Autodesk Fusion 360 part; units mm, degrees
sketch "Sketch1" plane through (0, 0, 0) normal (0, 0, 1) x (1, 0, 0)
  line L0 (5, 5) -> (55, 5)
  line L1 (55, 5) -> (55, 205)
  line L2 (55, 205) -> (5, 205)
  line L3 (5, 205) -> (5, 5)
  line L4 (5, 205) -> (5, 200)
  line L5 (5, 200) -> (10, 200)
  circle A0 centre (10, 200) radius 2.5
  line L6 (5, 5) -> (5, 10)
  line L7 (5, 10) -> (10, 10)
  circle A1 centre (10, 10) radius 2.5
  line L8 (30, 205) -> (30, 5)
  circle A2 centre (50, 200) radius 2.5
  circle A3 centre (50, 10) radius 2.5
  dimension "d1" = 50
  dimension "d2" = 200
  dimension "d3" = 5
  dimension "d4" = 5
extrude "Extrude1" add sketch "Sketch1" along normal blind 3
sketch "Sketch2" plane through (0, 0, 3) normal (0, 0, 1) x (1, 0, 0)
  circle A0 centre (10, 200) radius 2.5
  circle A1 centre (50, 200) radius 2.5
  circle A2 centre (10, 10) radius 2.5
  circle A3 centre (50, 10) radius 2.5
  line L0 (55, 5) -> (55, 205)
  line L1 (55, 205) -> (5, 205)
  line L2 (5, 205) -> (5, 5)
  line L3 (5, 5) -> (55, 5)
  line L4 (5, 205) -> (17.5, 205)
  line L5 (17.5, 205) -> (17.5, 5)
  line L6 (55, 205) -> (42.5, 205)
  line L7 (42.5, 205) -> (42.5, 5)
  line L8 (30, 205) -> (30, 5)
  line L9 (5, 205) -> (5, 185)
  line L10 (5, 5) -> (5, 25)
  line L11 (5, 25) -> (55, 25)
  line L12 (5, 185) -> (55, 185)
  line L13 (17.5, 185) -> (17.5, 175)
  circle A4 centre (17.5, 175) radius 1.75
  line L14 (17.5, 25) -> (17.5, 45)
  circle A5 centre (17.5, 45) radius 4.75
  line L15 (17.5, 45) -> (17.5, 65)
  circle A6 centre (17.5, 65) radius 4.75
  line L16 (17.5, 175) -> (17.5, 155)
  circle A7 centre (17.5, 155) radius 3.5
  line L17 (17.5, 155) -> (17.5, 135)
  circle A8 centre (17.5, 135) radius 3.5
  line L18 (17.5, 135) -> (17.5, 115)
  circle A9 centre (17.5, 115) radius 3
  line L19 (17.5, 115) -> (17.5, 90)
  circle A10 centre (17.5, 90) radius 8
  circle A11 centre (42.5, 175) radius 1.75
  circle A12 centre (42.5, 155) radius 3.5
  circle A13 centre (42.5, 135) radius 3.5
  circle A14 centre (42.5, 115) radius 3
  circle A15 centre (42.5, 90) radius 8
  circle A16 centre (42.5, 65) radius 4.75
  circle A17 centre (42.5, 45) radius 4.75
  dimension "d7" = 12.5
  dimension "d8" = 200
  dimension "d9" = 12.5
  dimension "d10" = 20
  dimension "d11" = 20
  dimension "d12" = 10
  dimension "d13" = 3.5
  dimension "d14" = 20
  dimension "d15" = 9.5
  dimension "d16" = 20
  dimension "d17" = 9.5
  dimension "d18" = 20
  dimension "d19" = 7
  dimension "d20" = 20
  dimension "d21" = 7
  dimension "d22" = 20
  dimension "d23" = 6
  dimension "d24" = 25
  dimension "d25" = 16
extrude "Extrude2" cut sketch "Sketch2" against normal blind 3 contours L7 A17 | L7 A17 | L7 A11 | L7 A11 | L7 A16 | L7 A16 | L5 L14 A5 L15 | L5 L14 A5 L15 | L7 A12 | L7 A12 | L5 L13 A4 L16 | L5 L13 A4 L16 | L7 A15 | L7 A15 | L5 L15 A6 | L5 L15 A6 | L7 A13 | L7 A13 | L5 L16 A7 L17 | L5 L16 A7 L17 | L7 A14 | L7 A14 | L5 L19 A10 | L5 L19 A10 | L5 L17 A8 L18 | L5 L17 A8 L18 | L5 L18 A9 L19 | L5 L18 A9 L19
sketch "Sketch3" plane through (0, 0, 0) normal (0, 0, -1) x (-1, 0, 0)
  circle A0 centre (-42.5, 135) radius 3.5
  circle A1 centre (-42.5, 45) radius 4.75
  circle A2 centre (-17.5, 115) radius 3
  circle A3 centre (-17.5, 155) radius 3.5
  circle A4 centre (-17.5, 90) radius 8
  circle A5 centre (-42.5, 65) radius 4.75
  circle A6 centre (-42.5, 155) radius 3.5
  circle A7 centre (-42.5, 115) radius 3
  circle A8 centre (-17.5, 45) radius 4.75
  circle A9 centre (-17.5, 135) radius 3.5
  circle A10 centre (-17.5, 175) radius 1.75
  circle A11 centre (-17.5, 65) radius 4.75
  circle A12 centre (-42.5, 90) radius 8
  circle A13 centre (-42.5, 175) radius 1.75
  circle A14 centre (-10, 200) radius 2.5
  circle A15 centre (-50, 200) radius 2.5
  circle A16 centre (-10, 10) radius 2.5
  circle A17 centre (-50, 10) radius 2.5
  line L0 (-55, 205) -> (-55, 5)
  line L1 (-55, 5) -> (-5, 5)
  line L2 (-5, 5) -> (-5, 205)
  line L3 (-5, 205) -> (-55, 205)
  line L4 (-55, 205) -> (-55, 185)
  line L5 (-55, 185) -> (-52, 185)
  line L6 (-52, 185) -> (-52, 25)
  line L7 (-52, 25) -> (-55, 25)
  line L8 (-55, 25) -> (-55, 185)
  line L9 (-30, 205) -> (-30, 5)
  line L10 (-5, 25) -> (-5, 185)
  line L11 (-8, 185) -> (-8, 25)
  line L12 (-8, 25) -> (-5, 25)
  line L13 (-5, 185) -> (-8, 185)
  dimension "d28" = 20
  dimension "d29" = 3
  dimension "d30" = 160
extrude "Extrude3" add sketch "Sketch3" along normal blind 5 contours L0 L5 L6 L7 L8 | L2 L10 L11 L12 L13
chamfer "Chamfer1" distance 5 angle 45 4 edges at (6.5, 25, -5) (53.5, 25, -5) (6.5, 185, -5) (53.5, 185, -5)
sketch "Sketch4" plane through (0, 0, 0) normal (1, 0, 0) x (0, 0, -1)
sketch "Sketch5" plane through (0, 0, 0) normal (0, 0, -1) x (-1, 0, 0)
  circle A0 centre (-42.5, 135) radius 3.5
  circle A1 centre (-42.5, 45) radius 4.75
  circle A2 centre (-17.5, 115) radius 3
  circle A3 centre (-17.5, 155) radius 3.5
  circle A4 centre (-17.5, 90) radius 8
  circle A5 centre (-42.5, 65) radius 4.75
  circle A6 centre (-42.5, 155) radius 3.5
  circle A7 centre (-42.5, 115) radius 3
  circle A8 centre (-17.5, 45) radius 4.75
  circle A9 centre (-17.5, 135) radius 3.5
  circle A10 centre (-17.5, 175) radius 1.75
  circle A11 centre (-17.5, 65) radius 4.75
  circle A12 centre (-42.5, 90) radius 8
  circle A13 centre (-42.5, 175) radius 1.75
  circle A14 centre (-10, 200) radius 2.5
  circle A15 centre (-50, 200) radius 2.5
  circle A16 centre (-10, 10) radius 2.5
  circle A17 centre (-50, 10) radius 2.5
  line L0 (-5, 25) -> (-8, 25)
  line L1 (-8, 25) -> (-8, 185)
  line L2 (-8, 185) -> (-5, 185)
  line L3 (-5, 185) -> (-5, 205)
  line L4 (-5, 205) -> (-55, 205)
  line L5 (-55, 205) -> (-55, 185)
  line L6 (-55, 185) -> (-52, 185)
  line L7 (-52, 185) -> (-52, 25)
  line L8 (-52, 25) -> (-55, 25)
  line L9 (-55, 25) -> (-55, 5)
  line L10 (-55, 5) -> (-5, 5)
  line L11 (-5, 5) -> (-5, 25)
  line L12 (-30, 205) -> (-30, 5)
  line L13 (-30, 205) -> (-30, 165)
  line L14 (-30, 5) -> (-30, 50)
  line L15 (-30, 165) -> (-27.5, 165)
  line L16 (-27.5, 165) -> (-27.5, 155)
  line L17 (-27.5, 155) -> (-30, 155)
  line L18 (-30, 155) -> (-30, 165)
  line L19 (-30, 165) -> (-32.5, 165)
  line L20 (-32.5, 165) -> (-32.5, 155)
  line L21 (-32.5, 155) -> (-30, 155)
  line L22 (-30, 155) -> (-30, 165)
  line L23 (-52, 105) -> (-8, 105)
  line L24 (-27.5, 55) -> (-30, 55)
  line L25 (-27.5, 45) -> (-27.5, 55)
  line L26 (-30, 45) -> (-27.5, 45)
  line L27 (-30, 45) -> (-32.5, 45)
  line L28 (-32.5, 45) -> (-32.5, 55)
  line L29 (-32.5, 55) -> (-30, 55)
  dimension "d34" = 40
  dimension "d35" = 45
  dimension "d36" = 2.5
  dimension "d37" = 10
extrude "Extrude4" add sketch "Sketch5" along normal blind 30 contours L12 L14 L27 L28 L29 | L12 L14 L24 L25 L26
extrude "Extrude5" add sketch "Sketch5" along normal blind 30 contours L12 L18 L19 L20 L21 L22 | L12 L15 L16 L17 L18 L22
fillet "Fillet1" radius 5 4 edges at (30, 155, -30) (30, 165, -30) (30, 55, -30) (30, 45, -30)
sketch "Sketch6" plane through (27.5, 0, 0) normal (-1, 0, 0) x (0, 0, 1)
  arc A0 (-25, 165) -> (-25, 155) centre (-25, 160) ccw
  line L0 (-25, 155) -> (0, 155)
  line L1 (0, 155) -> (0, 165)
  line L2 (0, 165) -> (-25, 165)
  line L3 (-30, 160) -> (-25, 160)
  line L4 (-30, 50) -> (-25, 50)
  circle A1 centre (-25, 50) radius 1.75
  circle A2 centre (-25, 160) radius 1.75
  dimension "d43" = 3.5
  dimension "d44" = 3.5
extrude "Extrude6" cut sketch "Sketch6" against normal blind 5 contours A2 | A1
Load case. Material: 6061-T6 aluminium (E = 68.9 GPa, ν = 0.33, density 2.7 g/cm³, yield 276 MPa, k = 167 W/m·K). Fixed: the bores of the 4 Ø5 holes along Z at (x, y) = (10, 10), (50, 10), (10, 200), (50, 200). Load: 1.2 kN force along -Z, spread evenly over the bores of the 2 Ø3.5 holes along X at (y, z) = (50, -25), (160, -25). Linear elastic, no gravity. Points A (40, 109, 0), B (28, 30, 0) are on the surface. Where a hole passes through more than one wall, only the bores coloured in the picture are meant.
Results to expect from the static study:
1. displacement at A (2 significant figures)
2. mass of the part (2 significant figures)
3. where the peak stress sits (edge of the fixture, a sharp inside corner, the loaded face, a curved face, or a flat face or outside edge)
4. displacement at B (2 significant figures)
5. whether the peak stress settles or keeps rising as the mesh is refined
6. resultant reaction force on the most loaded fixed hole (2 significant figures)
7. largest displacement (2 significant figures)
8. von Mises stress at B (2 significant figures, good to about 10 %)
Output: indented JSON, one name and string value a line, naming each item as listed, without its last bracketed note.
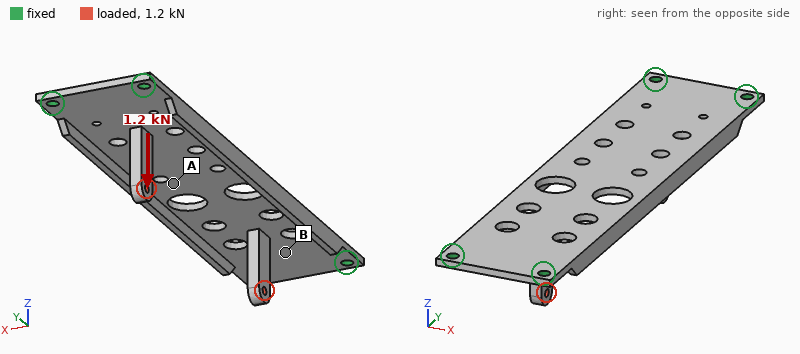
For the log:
{
  "displacement at A": "1.0 mm",
  "mass of the part": "93 g",
  "where the peak stress sits": "edge of the fixture",
  "displacement at B": "0.28 mm",
  "whether the peak stress settles or keeps rising as the mesh is refined": "keeps rising",
  "resultant reaction force on the most loaded fixed hole": "790 N",
  "largest displacement": "1.0 mm",
  "von Mises stress at B": "44 MPa"
}
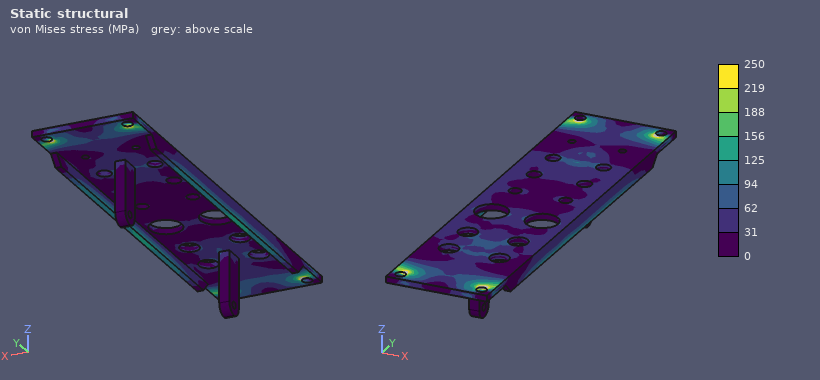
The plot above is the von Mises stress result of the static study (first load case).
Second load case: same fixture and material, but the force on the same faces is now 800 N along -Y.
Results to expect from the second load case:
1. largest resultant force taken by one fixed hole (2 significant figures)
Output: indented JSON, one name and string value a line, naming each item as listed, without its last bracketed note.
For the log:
{
  "largest resultant force taken by one fixed hole": "240 N"
}
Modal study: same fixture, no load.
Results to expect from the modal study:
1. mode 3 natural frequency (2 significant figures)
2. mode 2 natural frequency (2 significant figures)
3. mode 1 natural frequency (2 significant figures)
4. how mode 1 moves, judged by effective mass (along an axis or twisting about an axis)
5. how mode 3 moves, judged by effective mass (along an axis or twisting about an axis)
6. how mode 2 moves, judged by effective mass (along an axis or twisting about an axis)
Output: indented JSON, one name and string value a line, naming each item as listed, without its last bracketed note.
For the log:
{
  "mode 3 natural frequency": "1700 Hz",
  "mode 2 natural frequency": "1100 Hz",
  "mode 1 natural frequency": "610 Hz",
  "how mode 1 moves, judged by effective mass": "along Z",
  "how mode 3 moves, judged by effective mass": "twisting about X",
  "how mode 2 moves, judged by effective mass": "twisting about Y"
}
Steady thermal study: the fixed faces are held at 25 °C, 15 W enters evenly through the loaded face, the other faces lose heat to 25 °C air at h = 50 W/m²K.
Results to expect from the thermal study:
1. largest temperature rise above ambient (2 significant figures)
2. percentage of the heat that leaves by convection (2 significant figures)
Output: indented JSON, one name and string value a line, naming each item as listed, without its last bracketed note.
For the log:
{
  "largest temperature rise above ambient": "32 K",
  "percentage of the heat that leaves by convection": "49 %"
}
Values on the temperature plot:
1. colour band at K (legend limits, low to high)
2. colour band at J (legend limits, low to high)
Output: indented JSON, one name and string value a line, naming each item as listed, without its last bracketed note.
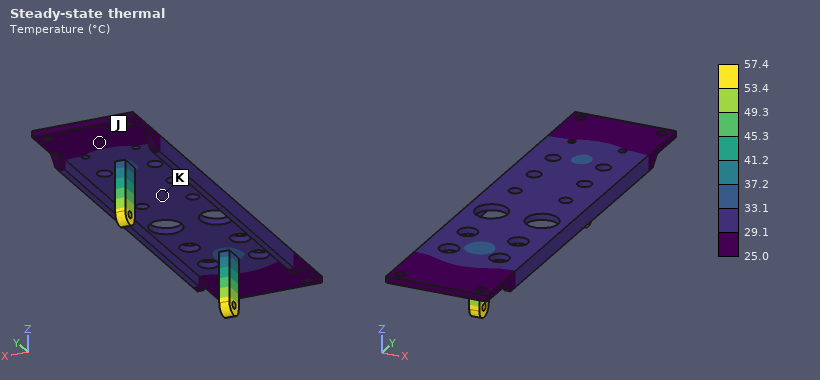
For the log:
{
  "colour band at K": "29.1 to 33.1 °C",
  "colour band at J": "25.0 to 29.1 °C"
}
